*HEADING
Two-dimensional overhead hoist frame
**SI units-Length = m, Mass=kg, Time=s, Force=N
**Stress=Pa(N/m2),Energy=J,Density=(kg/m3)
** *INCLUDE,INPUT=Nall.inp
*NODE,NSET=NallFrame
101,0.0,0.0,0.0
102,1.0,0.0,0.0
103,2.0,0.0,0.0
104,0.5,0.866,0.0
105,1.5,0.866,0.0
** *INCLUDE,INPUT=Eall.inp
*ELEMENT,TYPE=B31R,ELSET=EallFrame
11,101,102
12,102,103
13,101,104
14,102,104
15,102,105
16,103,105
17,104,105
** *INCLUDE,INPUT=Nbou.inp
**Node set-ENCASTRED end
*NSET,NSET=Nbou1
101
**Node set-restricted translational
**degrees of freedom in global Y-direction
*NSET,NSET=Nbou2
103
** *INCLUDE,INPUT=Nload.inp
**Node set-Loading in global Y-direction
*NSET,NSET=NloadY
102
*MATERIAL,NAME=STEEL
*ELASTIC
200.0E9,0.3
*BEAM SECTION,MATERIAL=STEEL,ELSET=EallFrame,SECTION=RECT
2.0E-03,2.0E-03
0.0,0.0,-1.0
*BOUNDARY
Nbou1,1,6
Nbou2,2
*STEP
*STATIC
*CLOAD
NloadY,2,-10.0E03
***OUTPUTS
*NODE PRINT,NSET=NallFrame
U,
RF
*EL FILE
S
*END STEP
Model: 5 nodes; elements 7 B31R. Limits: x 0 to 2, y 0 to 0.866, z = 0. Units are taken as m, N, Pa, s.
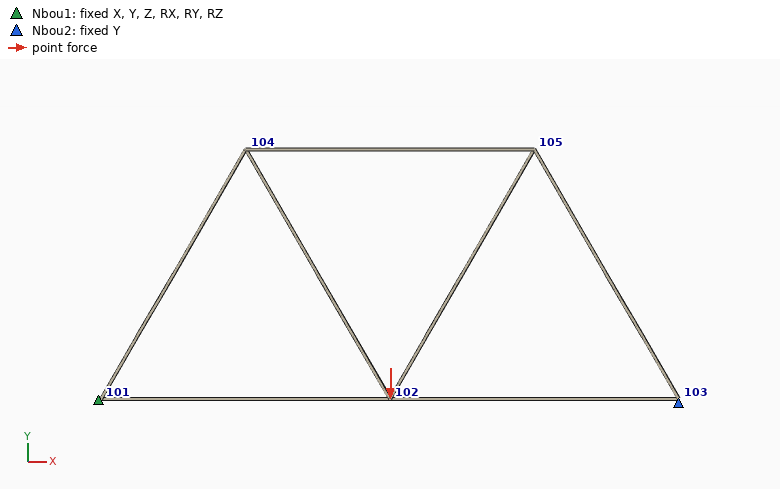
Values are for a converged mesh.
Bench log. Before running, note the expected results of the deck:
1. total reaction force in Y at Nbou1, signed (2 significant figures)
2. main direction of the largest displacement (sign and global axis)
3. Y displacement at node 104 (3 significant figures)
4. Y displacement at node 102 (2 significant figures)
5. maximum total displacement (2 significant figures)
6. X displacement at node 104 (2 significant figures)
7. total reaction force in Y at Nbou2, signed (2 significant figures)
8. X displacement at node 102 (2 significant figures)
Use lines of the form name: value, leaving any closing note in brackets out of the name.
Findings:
total reaction force in Y at Nbou1, signed: 5000 N
main direction of the largest displacement: -Y
Y displacement at node 104: -0.0125 m
Y displacement at node 102: -0.023 m
maximum total displacement: 0.023 m
X displacement at node 104: 0.0072 m
total reaction force in Y at Nbou2, signed: 5000 N
X displacement at node 102: 0.0036 m
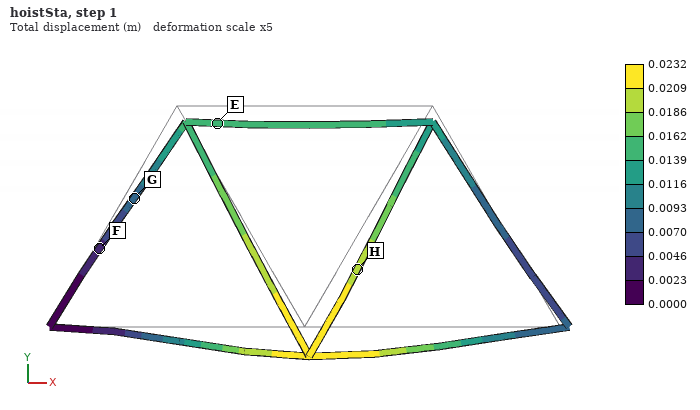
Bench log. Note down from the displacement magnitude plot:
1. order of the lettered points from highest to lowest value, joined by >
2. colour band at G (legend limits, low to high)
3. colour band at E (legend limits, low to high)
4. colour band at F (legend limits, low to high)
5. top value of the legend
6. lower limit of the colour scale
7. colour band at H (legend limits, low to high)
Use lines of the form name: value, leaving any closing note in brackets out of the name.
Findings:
order of the lettered points from highest to lowest value, joined by >: H > E > G > F
colour band at G: 0.0070 to 0.0093 m
colour band at E: 0.0139 to 0.0162 m
colour band at F: 0.0023 to 0.0046 m
top value of the legend: 0.0232 m
lower limit of the colour scale: 0.0000 m
colour band at H: 0.0186 to 0.0209 m
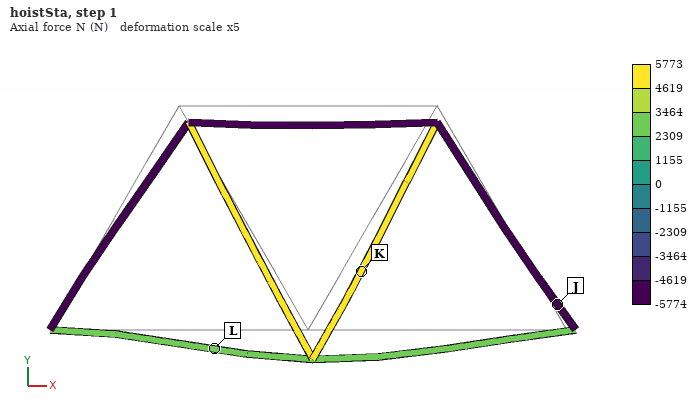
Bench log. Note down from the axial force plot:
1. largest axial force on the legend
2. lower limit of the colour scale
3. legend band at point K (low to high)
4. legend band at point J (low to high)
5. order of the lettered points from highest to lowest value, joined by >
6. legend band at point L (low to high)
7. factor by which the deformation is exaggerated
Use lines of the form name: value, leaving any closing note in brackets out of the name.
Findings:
largest axial force on the legend: 5773 N
lower limit of the colour scale: -5774 N
legend band at point K: 4619 to 5773 N
legend band at point J: -5774 to -4619 N
order of the lettered points from highest to lowest value, joined by >: K > L > J
legend band at point L: 2309 to 3464 N
factor by which the deformation is exaggerated: 5
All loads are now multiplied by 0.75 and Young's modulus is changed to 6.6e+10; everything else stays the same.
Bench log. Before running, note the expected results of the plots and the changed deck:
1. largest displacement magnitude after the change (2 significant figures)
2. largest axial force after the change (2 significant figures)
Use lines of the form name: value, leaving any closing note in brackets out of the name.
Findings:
largest displacement magnitude after the change: 0.053 m
largest axial force after the change: 4300 N
